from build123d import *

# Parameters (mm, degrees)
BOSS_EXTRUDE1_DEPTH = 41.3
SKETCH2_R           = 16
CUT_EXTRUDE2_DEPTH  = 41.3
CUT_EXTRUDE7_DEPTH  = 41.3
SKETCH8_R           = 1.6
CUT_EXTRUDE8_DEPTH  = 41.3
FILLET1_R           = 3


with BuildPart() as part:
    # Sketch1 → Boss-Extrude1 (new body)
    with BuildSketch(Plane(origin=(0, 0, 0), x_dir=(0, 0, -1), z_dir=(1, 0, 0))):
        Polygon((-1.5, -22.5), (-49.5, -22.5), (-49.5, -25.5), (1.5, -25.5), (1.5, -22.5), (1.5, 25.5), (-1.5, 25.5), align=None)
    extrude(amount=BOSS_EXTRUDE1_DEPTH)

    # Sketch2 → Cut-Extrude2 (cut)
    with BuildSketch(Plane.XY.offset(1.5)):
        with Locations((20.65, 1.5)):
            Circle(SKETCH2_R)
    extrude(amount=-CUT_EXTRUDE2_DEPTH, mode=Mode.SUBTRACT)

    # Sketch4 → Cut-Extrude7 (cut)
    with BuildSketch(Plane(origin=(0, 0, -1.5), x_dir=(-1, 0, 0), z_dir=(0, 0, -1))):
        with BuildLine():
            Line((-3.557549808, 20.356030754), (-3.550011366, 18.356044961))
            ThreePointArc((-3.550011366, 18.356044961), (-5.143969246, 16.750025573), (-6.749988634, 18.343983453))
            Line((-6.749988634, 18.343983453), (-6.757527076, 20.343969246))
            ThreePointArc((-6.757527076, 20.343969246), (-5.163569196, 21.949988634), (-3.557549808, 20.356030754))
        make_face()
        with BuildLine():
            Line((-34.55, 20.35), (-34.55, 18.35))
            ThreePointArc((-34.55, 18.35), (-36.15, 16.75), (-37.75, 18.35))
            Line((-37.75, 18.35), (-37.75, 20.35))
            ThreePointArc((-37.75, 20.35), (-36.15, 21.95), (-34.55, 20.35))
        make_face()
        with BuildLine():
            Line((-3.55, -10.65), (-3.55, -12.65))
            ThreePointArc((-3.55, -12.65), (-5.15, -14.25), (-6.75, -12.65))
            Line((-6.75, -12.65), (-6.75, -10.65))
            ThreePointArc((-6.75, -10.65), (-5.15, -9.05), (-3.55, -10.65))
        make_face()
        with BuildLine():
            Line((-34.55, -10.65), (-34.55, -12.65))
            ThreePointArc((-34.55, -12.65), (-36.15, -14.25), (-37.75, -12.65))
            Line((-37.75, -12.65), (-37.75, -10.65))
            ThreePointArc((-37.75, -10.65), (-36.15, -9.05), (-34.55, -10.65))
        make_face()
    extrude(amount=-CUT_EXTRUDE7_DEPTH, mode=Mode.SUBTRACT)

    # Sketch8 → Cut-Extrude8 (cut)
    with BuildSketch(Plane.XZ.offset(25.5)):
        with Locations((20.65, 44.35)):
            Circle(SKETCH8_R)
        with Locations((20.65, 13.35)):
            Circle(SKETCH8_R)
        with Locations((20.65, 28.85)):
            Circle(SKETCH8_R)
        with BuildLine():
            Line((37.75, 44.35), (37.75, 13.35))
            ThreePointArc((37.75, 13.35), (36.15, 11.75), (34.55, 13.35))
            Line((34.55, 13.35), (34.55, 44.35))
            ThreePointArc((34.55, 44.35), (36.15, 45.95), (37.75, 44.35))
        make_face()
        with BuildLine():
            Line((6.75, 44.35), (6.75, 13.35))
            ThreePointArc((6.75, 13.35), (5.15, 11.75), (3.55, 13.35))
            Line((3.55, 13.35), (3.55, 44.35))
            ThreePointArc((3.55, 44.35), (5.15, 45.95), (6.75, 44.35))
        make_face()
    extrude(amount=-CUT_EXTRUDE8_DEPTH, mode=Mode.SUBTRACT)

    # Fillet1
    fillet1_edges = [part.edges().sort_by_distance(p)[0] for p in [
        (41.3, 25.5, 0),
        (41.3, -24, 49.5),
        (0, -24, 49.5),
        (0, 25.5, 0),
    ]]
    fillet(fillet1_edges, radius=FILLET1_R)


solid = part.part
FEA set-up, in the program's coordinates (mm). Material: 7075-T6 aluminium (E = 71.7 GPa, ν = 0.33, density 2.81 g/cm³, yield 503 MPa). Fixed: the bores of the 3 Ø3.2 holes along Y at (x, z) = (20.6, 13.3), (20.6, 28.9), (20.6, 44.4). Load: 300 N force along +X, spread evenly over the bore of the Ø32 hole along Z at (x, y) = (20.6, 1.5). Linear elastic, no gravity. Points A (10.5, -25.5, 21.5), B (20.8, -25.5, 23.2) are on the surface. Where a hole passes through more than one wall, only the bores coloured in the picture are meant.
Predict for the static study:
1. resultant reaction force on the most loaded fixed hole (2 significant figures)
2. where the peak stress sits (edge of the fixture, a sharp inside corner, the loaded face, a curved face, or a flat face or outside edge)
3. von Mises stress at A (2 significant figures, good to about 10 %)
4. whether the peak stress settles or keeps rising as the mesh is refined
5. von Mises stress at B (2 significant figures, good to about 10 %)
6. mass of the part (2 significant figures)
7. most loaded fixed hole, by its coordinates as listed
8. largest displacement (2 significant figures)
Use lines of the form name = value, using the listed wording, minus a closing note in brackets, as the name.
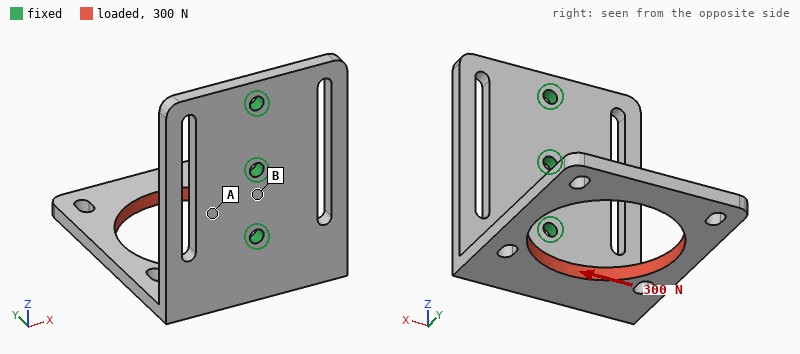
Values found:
resultant reaction force on the most loaded fixed hole = 430 N
where the peak stress sits = edge of the fixture
von Mises stress at A = 58 MPa
whether the peak stress settles or keeps rising as the mesh is refined = keeps rising
von Mises stress at B = 22 MPa
mass of the part = 25 g
most loaded fixed hole, by its coordinates as listed = (20.6, 13.3)
largest displacement = 0.69 mm
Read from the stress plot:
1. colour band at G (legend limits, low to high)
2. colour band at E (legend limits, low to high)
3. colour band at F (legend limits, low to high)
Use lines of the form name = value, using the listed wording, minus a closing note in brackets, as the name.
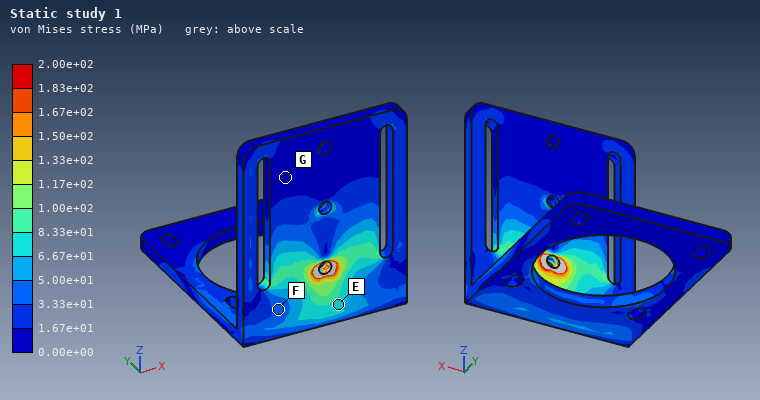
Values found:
colour band at G = 0.00e+00 to 1.67e+01 MPa
colour band at E = 6.67e+01 to 8.33e+01 MPa
colour band at F = 3.33e+01 to 5.00e+01 MPa
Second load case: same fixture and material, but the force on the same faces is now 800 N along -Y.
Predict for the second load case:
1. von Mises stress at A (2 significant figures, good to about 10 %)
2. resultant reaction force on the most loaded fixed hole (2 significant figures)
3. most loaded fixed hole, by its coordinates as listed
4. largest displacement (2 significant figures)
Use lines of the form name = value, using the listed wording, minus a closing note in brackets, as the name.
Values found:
von Mises stress at A = 34 MPa
resultant reaction force on the most loaded fixed hole = 1.1 kN
most loaded fixed hole, by its coordinates as listed = (20.6, 13.3)
largest displacement = 0.72 mm
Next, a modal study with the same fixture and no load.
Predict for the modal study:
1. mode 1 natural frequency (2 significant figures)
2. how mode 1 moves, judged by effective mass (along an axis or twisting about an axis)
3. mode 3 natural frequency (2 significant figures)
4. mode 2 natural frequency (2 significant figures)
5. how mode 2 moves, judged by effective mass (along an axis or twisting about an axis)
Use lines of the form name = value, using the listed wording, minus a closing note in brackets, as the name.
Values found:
mode 1 natural frequency = 660 Hz
how mode 1 moves, judged by effective mass = along Z
mode 3 natural frequency = 2000 Hz
mode 2 natural frequency = 1200 Hz
how mode 2 moves, judged by effective mass = along X
